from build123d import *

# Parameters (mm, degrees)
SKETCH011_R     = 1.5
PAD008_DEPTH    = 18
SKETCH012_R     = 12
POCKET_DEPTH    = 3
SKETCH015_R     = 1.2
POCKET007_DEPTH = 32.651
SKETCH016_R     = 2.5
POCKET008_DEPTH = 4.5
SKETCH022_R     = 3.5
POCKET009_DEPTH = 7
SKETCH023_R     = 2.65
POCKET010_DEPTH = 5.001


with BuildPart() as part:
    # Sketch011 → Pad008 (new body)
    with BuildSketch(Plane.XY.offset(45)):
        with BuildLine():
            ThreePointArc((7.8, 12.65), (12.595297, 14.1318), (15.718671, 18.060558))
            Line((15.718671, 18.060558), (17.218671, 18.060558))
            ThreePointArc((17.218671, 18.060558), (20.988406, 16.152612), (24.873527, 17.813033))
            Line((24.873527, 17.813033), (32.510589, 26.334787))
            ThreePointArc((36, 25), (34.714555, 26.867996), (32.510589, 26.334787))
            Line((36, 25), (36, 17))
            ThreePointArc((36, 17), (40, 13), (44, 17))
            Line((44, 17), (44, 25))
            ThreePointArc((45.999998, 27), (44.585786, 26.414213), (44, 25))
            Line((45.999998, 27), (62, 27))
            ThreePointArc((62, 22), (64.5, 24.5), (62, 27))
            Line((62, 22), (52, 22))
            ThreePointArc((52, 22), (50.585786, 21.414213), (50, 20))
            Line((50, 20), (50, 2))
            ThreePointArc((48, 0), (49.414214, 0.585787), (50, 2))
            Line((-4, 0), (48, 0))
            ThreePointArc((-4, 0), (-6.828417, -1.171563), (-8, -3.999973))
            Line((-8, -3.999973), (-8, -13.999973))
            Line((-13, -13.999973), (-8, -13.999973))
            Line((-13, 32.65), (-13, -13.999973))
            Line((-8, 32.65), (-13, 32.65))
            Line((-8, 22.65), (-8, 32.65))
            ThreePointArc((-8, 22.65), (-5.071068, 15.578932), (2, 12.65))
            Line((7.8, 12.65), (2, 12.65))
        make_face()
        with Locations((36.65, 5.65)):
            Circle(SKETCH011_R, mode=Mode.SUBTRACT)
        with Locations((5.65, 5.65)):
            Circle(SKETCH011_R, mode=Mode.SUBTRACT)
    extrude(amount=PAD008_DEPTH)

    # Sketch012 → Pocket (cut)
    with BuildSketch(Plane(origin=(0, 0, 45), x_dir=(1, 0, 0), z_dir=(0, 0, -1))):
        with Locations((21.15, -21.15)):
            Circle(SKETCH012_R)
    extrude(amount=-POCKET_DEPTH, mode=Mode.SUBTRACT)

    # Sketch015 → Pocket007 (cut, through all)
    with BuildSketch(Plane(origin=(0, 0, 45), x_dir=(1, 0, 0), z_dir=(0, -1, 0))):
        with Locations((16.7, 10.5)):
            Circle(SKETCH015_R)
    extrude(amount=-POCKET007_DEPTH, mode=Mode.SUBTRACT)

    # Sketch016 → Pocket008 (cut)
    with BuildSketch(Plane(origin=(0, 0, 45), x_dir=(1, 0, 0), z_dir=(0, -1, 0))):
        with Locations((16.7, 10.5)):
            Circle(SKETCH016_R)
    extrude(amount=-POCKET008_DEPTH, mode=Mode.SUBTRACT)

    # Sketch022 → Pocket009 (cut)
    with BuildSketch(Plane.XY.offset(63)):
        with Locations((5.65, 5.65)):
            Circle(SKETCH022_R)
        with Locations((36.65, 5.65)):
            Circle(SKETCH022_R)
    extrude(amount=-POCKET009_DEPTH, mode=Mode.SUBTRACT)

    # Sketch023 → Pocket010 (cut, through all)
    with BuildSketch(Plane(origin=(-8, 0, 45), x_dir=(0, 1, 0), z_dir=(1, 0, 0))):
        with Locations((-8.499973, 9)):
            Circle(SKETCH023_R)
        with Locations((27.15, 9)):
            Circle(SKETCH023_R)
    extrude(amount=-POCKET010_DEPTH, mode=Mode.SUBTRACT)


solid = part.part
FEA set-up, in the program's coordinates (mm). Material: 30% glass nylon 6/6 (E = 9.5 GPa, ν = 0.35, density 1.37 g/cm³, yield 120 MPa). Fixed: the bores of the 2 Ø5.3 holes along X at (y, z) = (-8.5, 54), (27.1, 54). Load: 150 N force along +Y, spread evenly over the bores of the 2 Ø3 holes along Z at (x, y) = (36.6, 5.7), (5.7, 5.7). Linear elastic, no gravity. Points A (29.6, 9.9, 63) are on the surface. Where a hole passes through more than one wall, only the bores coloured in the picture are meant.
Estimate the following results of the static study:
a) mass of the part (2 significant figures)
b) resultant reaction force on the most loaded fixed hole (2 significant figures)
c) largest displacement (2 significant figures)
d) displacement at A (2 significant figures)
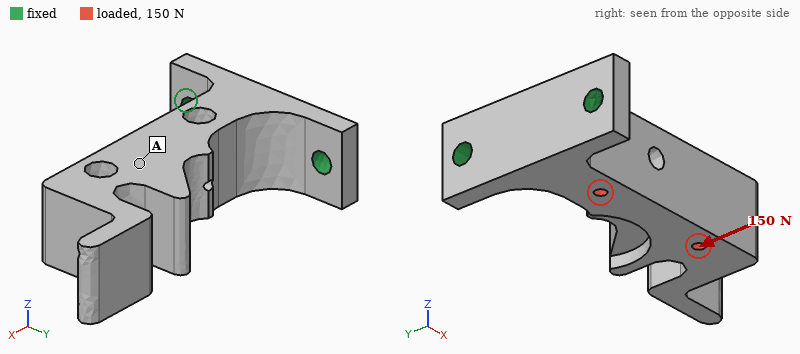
31 g
200 N
0.23 mm
0.099 mm
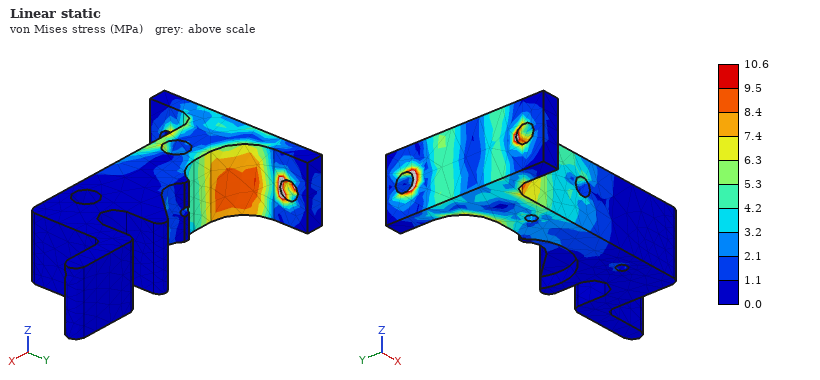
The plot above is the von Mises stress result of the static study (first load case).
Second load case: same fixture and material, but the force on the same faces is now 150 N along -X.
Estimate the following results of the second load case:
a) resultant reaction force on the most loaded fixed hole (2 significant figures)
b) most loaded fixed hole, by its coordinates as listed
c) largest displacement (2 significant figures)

100 N
(-8.5, 54)
68 µm
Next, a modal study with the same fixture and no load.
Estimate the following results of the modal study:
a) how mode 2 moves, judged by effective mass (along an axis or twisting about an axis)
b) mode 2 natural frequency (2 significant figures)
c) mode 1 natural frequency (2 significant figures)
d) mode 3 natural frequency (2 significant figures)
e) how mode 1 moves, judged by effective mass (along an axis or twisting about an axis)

along Y
910 Hz
590 Hz
3200 Hz
along Z
